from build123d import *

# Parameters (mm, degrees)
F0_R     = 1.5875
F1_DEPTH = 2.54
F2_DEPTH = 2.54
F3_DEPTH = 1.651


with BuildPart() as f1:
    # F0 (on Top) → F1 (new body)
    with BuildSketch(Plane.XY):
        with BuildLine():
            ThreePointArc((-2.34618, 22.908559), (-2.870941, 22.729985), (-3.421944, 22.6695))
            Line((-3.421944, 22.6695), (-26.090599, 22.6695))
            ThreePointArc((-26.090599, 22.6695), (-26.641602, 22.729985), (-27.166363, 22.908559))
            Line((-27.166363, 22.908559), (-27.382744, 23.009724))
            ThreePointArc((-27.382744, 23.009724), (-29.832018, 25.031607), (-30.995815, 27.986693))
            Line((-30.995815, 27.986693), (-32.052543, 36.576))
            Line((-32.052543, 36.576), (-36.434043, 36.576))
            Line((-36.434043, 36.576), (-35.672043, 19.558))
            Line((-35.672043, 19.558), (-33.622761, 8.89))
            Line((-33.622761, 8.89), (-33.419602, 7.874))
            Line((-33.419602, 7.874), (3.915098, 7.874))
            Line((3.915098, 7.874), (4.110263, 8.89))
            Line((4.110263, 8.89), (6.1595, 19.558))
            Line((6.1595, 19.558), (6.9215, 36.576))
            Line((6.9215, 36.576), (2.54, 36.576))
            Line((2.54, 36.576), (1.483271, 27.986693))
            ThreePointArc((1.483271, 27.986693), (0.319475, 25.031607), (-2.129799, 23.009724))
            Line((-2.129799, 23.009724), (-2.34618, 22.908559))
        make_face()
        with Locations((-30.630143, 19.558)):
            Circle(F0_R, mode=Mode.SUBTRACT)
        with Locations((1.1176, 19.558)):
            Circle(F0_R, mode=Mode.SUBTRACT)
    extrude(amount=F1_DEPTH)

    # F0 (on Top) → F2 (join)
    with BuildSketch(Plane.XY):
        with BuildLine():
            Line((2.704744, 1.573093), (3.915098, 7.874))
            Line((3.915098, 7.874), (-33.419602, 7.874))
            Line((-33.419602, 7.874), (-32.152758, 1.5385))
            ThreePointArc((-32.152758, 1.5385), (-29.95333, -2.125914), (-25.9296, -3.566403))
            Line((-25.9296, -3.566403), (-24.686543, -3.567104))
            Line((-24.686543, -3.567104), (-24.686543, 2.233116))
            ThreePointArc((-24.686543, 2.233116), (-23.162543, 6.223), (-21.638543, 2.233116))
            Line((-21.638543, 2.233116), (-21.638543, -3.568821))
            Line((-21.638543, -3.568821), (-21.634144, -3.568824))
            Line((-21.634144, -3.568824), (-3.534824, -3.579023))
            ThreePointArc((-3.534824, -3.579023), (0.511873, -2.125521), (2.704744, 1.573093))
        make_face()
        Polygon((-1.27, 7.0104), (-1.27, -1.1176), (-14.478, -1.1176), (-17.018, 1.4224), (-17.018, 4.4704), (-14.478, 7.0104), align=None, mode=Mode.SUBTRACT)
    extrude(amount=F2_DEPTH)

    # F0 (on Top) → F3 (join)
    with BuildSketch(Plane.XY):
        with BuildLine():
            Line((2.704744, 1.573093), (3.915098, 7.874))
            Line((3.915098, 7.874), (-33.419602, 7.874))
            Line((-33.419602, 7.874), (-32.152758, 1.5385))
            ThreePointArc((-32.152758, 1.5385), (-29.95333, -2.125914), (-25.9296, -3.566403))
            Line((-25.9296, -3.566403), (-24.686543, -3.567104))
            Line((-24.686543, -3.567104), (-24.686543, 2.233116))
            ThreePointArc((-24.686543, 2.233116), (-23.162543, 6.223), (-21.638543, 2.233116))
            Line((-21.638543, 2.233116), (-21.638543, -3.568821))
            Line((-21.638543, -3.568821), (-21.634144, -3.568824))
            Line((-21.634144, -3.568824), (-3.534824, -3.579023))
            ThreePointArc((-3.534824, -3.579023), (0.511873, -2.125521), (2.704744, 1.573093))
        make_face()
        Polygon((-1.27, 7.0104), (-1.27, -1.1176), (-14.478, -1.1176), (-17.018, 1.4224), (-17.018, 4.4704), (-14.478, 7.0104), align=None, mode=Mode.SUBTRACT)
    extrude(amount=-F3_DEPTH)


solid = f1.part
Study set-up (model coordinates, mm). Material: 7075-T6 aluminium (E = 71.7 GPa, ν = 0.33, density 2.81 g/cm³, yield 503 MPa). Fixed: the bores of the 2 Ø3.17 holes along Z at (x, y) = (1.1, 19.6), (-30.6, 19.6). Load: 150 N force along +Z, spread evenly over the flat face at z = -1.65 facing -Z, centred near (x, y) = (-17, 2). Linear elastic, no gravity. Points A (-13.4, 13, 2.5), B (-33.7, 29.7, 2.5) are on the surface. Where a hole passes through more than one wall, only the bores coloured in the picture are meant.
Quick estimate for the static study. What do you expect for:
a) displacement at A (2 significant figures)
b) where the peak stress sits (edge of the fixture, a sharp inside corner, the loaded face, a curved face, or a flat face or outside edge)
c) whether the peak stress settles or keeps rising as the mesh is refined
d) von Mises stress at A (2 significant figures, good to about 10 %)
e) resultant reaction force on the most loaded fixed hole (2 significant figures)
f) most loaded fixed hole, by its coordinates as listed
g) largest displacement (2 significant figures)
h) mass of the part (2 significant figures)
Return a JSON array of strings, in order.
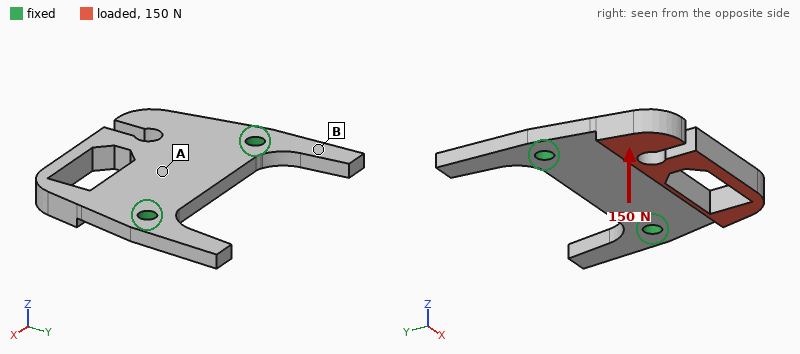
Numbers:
["0.030 mm", "edge of the fixture", "keeps rising", "24 MPa", "84 N", "(-30.6, 19.6)", "0.15 mm", "8.0 g"]
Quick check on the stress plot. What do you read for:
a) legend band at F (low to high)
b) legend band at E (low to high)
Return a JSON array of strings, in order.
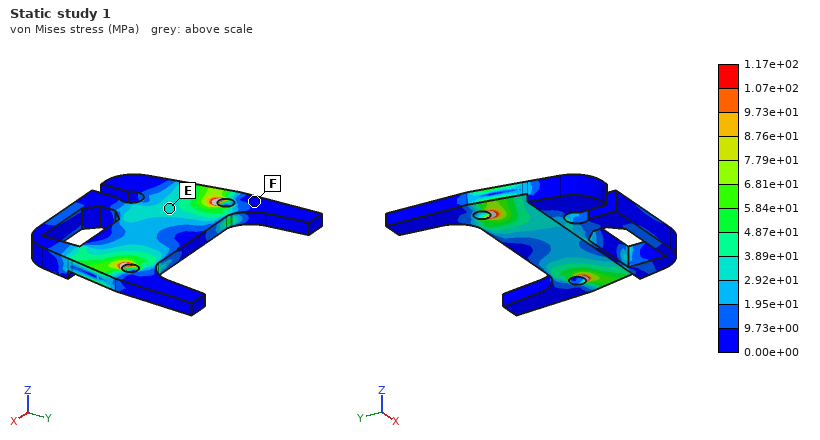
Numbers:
["0.00e+00 to 9.73e+00 MPa", "2.92e+01 to 3.89e+01 MPa"]
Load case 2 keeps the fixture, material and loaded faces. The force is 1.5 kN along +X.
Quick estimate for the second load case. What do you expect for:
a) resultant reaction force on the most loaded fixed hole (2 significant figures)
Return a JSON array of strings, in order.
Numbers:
["1.1 kN"]
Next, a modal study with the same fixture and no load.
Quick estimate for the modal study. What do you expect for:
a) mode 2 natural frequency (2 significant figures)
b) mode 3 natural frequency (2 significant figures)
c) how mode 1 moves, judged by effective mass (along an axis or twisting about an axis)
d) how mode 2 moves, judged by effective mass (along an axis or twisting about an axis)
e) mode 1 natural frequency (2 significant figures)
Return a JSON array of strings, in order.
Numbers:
["6700 Hz", "9000 Hz", "along Z", "twisting about Y", "3400 Hz"]
